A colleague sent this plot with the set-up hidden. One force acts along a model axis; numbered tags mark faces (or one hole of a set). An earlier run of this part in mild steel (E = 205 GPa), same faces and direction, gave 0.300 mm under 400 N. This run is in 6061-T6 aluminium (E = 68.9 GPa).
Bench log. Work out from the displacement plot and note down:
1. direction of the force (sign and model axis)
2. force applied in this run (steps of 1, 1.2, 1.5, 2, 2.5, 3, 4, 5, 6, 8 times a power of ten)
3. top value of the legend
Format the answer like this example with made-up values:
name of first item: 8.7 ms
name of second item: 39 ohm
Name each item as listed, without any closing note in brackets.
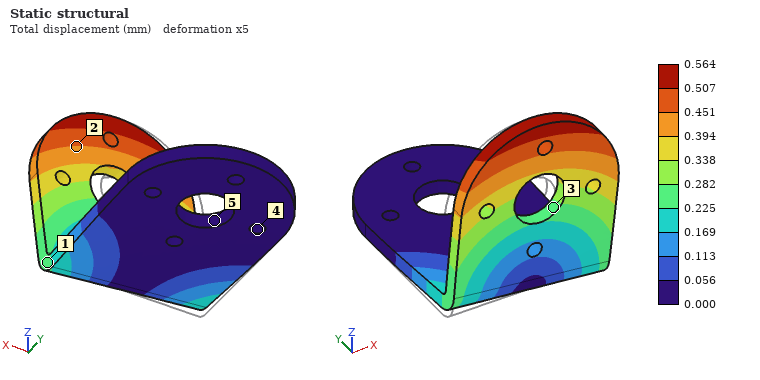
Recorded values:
direction of the force: +X
force applied in this run: 250 N
top value of the legend: 0.564 mm
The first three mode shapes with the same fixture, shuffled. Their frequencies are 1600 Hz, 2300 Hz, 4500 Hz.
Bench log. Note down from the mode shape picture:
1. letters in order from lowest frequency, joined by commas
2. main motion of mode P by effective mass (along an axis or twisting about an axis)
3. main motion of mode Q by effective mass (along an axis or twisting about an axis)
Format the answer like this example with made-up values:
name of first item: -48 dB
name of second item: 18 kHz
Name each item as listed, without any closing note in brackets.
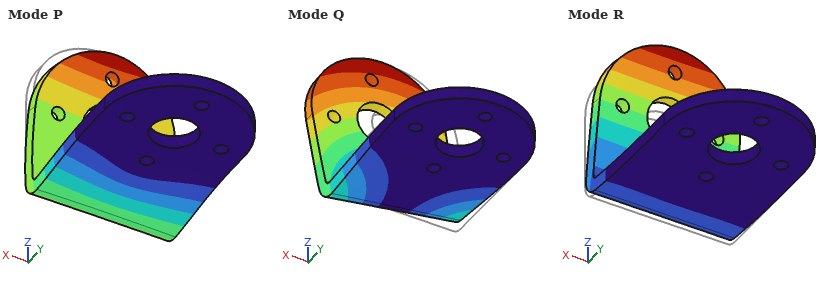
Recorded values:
letters in order from lowest frequency, joined by commas: R, Q, P
main motion of mode P by effective mass: along Z
main motion of mode Q by effective mass: along X
